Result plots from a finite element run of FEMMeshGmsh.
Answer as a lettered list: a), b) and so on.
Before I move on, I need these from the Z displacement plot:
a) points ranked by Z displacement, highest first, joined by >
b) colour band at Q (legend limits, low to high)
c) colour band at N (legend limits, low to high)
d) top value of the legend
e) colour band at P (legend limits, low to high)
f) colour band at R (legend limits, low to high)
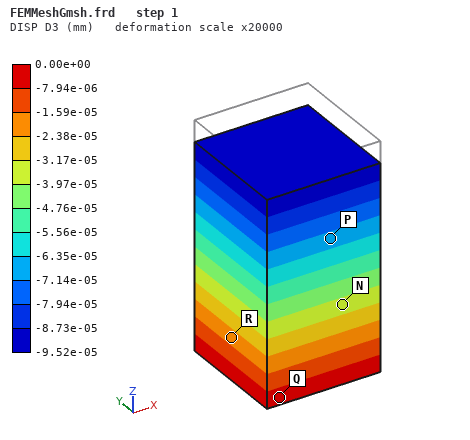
a) Q > R > N > P
b) -7.94e-06 to 0.00e+00 mm
c) -3.97e-05 to -3.17e-05 mm
d) 0.00e+00 mm
e) -7.14e-05 to -6.35e-05 mm
f) -2.38e-05 to -1.59e-05 mm
